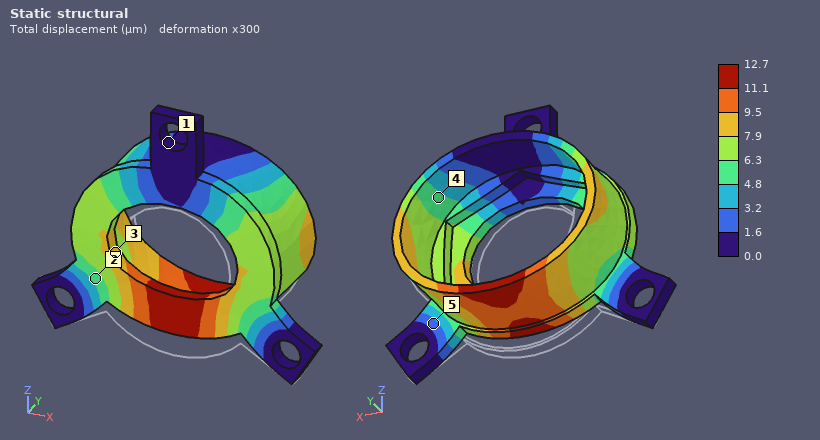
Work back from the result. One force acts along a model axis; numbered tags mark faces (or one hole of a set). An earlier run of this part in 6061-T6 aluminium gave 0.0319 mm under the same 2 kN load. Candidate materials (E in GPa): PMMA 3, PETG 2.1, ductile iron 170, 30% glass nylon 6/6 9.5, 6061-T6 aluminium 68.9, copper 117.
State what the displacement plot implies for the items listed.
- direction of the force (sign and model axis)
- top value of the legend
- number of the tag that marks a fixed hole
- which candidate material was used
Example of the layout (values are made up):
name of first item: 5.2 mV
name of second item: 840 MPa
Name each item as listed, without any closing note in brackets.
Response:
direction of the force: +Z
top value of the legend: 12.7 µm
number of the tag that marks a fixed hole: 1
which candidate material was used: ductile iron
